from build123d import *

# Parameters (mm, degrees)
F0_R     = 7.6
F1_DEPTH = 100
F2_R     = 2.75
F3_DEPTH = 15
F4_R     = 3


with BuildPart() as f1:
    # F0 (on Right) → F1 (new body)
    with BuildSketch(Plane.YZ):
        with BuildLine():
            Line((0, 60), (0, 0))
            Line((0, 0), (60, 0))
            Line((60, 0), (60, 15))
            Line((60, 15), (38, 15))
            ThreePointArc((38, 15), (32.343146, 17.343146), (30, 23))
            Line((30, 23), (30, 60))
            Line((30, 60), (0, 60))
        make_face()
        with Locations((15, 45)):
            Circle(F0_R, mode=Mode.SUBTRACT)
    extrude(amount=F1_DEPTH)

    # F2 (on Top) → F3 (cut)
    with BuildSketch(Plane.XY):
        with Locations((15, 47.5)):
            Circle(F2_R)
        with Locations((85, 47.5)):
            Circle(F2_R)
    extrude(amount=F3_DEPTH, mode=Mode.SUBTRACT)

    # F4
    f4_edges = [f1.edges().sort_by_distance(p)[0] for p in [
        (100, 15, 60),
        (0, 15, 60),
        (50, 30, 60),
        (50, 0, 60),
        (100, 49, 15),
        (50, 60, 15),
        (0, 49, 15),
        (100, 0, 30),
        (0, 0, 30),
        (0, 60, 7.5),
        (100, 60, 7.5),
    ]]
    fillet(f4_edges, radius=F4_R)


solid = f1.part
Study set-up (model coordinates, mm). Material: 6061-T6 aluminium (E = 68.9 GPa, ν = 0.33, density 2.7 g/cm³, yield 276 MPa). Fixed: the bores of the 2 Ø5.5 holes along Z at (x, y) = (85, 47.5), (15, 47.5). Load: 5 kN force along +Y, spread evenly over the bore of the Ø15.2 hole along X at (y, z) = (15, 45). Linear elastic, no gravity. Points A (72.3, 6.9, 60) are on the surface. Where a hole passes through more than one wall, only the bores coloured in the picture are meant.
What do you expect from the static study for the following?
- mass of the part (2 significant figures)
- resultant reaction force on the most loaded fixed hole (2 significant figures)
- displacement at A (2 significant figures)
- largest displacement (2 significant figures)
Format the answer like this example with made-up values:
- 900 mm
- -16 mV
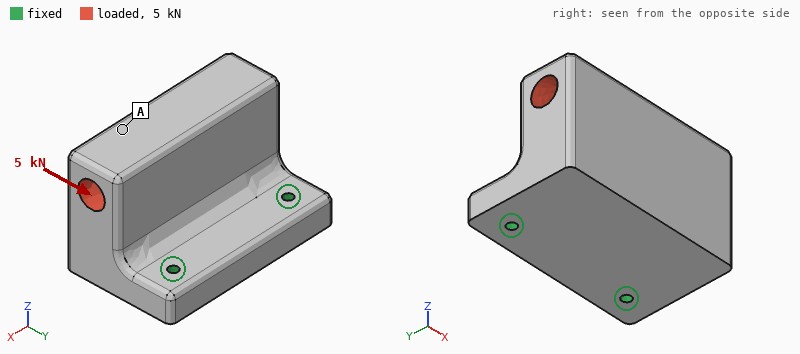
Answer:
- 560 g
- 2.6 kN
- 0.19 mm
- 0.20 mm
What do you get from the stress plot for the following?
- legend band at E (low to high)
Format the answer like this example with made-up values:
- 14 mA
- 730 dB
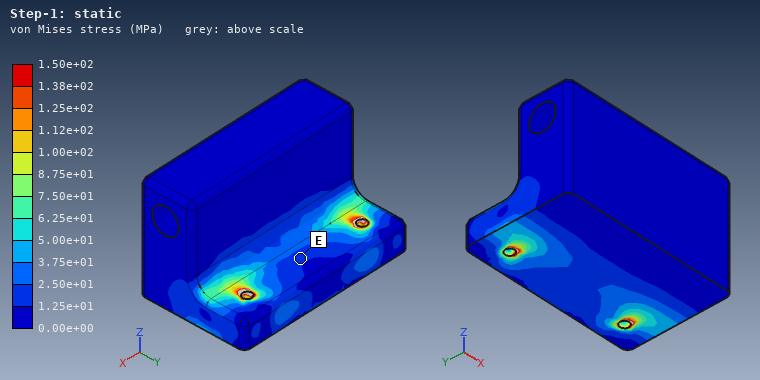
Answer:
- 1.25e+01 to 2.50e+01 MPa
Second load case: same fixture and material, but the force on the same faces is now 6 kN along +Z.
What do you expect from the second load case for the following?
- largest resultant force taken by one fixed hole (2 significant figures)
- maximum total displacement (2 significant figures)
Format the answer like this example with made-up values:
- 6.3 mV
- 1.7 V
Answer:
- 3.0 kN
- 0.16 mm
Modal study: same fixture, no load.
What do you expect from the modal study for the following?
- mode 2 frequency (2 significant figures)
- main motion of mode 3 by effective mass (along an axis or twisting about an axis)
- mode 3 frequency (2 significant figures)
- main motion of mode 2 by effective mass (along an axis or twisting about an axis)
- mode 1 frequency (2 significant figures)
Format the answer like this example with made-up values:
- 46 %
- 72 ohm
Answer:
- 4100 Hz
- along X
- 6500 Hz
- along X
- 1600 Hz
